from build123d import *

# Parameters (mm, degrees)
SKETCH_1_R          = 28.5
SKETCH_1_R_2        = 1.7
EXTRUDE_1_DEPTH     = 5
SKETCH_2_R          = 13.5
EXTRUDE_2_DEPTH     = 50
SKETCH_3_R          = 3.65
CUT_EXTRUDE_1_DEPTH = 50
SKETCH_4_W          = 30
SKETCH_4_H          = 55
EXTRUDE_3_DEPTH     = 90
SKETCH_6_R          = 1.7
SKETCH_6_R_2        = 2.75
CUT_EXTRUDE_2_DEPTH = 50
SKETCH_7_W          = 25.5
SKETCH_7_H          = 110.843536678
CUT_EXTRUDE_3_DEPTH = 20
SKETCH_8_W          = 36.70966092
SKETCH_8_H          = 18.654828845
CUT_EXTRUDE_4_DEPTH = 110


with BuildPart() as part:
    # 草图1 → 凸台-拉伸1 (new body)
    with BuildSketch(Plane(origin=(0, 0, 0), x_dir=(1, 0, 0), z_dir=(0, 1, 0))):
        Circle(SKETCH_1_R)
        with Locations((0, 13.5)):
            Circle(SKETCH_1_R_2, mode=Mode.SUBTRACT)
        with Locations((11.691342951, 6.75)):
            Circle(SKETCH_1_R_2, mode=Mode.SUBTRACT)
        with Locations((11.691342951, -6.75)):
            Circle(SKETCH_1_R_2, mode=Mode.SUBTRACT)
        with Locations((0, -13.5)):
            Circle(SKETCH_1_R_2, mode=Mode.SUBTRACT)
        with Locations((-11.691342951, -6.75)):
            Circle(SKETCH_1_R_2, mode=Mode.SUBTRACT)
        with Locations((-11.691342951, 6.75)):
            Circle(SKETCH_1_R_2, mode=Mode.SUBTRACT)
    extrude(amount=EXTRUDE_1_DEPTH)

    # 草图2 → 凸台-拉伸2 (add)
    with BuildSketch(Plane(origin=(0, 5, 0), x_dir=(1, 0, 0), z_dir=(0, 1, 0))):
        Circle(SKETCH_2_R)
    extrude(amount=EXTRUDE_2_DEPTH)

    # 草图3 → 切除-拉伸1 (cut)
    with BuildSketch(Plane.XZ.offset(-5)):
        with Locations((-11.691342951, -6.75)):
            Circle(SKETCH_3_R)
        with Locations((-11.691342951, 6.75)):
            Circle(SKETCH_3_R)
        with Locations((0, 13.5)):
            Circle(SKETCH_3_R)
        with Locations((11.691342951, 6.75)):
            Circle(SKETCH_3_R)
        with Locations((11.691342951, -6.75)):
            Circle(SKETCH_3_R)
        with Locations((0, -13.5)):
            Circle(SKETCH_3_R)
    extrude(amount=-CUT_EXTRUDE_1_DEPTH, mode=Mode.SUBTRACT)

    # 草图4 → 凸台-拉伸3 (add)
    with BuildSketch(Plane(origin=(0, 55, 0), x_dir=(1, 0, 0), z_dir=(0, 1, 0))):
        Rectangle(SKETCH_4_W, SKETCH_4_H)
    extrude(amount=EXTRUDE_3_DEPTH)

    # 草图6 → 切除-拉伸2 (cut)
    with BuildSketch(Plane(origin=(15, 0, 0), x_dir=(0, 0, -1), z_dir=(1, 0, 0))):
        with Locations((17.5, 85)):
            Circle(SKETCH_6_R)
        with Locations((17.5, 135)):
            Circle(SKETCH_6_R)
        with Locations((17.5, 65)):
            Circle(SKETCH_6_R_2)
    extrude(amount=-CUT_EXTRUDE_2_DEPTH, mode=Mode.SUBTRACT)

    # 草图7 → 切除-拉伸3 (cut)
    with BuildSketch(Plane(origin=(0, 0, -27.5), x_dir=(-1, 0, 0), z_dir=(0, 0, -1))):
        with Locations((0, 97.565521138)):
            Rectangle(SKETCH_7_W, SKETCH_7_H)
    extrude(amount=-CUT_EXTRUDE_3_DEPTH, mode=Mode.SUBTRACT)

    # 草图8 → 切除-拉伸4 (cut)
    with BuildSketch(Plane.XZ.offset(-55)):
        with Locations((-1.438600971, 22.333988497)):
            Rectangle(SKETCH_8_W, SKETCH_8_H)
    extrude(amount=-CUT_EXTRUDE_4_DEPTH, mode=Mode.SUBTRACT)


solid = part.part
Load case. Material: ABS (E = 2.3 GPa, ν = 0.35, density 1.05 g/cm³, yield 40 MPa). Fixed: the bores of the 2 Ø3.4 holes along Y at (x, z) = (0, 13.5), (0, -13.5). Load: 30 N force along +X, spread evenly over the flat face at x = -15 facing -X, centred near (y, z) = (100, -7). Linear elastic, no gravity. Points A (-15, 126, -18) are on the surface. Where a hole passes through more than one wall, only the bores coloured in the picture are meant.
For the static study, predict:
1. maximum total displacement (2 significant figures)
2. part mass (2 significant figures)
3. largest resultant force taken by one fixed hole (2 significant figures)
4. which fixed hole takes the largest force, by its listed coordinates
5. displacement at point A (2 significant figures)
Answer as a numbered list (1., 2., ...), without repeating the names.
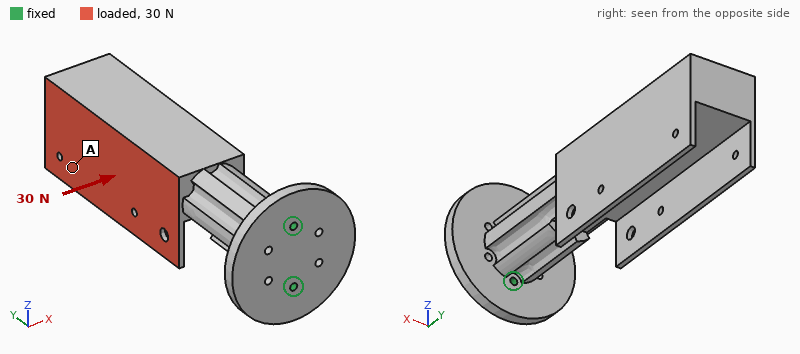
1. 1.9 mm
2. 100 g
3. 23 N
4. (0, -13.5)
5. 1.6 mm
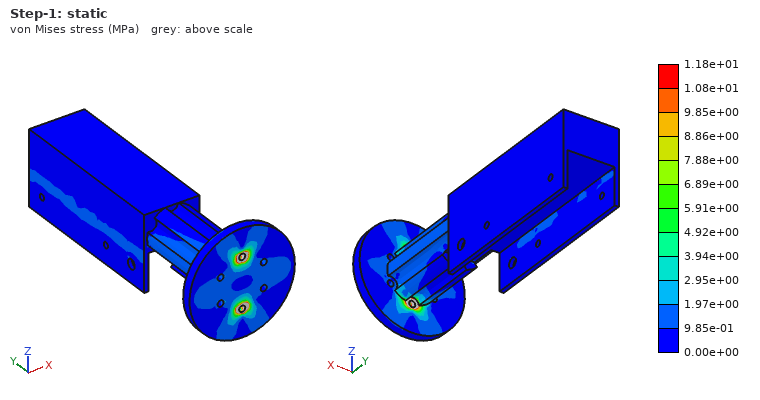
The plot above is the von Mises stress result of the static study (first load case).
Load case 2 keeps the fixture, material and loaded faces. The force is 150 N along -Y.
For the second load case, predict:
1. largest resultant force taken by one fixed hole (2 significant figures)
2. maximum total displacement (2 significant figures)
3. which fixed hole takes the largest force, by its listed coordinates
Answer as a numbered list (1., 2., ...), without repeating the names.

1. 120 N
2. 1.6 mm
3. (0, -13.5)
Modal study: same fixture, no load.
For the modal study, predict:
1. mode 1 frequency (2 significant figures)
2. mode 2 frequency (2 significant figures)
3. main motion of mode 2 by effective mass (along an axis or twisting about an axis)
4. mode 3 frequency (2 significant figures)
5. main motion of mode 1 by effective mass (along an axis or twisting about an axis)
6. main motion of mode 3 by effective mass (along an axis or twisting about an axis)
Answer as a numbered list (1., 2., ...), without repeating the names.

1. 93 Hz
2. 170 Hz
3. along Z
4. 740 Hz
5. along X
6. twisting about Y
